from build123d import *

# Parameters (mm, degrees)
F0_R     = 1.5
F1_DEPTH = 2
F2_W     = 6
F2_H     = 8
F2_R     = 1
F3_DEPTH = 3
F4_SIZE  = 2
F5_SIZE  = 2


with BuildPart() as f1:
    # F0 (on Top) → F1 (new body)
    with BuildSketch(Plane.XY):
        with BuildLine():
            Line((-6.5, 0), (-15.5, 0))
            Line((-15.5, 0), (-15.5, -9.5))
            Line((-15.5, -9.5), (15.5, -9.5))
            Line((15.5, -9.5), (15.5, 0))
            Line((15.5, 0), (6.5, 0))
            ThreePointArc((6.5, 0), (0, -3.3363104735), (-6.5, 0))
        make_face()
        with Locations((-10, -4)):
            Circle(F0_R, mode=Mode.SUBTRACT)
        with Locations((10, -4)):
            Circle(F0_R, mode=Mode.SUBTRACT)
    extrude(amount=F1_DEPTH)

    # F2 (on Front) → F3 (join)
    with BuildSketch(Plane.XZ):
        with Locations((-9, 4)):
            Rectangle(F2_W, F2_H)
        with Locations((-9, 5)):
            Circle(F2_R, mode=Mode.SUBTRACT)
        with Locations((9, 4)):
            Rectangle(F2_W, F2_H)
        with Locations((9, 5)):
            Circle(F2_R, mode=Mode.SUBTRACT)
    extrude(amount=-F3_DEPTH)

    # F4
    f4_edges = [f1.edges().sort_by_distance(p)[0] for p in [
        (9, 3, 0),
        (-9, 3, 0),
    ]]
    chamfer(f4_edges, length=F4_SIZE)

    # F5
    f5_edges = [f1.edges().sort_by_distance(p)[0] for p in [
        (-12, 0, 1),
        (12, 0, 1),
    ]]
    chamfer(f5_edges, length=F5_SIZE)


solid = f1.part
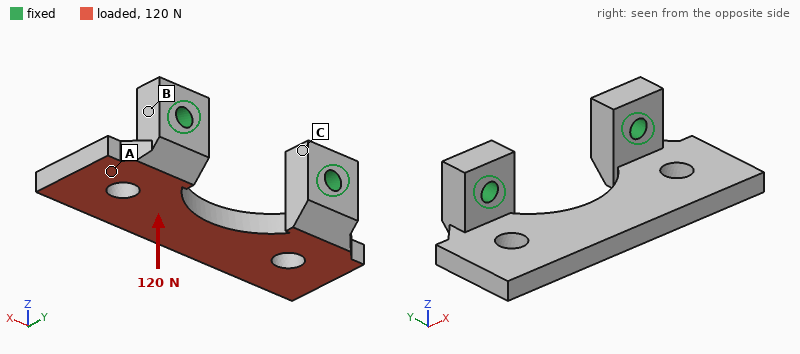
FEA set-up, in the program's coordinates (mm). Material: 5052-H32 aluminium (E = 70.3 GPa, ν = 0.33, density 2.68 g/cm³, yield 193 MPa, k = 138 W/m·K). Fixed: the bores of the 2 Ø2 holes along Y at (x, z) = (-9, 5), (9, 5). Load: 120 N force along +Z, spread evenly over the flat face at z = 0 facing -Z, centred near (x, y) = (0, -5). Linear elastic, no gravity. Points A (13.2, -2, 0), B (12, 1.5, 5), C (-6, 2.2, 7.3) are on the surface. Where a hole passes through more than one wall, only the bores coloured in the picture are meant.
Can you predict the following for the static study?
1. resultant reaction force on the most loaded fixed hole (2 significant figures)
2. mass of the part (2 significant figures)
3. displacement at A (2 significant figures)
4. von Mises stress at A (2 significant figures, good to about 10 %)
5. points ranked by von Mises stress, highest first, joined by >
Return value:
60 N
2.0 g
12 µm
26 MPa
A > B > C
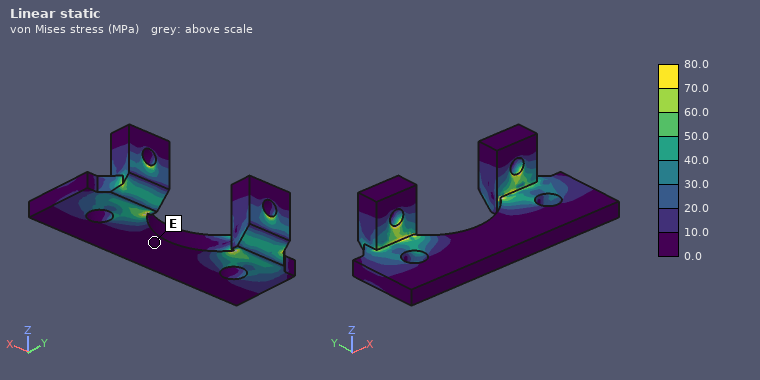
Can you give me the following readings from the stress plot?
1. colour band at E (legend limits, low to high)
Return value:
0.0 to 10.0 MPa
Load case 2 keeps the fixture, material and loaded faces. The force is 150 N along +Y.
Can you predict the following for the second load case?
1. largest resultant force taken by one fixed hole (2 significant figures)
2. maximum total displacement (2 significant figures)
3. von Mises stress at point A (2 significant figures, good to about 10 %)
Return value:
75 N
21 µm
11 MPa
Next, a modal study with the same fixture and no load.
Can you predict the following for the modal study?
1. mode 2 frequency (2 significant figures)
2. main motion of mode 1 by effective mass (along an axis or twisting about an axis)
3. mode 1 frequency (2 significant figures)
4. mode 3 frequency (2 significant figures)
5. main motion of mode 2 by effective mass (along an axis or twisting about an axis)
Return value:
12 kHz
along Z
8000 Hz
19 kHz
twisting about Y
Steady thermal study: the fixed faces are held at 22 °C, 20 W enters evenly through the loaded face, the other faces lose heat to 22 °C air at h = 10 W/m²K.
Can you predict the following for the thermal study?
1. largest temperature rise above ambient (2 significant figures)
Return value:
43 K
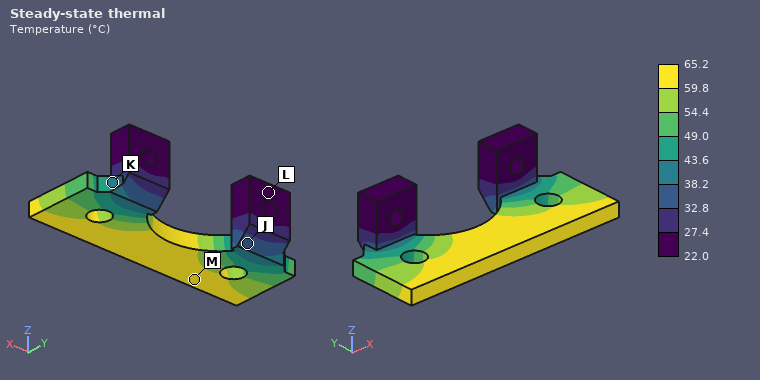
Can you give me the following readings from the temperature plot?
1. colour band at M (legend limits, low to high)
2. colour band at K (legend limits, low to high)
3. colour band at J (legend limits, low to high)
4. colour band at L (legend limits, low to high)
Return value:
59.8 to 65.2 °C
38.2 to 43.6 °C
32.8 to 38.2 °C
22.0 to 27.4 °C
